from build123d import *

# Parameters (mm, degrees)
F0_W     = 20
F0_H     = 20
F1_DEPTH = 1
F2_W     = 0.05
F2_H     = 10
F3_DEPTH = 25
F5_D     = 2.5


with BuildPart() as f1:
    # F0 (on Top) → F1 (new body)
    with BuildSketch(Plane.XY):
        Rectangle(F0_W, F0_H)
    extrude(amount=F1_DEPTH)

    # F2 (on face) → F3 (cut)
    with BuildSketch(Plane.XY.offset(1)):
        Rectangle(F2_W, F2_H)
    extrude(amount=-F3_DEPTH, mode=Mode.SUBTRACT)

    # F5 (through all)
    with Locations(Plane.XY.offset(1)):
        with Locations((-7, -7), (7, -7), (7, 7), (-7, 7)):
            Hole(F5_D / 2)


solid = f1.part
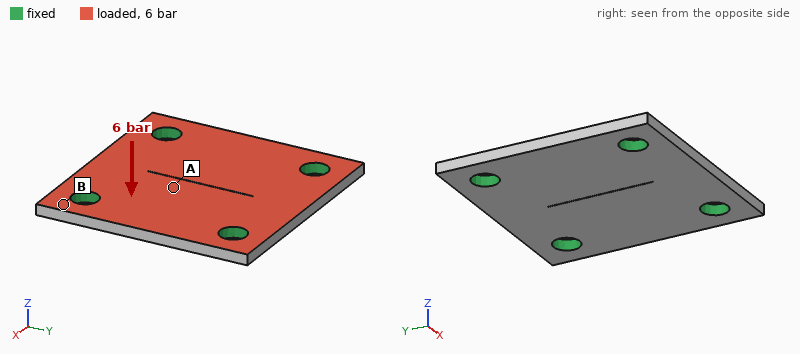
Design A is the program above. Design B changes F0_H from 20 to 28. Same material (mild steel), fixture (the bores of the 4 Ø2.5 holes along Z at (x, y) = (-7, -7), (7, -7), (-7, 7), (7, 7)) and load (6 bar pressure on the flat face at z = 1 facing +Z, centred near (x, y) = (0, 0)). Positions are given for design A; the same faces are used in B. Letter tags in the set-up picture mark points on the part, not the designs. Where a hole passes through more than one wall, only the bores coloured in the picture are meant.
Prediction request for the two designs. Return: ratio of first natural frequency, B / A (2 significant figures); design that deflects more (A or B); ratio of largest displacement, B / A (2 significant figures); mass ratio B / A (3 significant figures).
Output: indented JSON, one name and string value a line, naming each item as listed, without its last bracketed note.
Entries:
{
  "ratio of first natural frequency, B / A": "0.83",
  "design that deflects more": "B",
  "ratio of largest displacement, B / A": "1.3",
  "mass ratio B / A": "1.42"
}
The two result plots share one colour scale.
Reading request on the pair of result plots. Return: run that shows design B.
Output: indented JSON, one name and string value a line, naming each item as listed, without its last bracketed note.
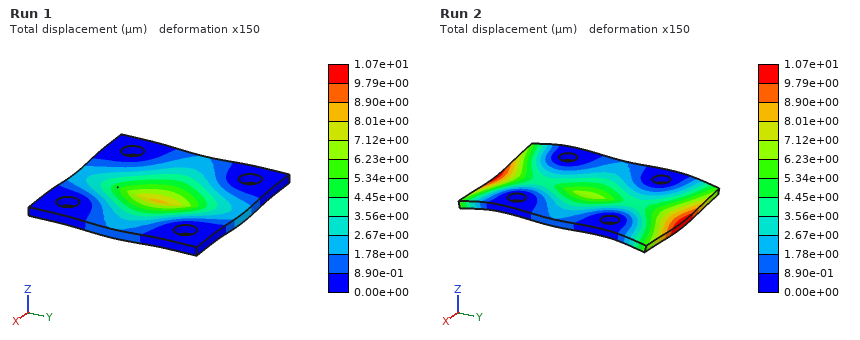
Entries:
{
  "run that shows design B": "Run 2"
}
